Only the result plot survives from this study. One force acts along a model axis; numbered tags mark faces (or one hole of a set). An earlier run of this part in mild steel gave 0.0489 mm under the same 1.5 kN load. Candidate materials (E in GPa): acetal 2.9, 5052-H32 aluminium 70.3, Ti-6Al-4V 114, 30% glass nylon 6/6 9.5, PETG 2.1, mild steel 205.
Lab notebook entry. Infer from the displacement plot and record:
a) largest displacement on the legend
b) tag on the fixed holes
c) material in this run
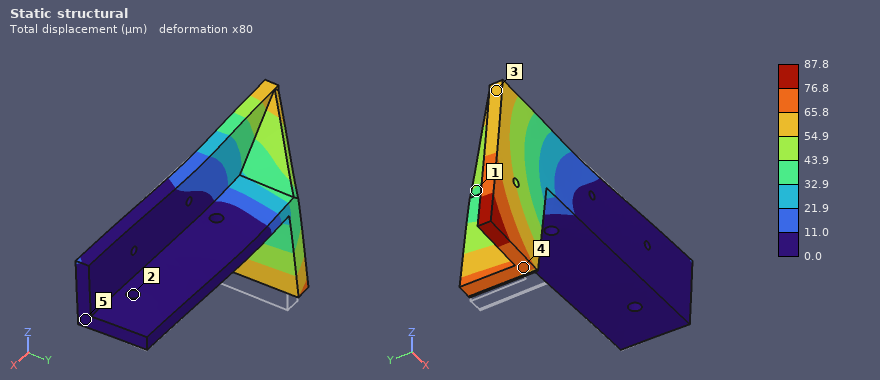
87.8 µm
2
Ti-6Al-4V
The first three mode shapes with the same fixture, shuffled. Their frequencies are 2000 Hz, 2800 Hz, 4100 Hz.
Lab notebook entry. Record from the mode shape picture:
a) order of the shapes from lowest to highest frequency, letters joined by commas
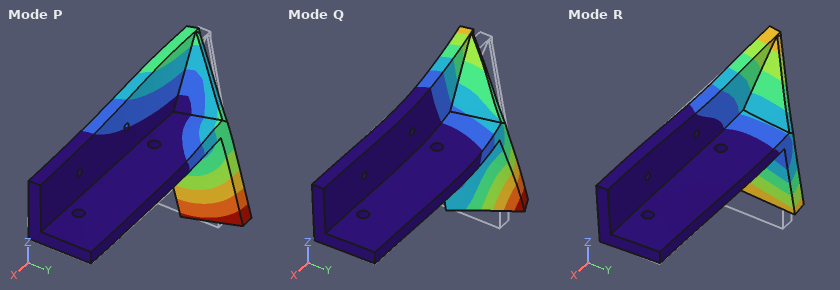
P, R, Q
